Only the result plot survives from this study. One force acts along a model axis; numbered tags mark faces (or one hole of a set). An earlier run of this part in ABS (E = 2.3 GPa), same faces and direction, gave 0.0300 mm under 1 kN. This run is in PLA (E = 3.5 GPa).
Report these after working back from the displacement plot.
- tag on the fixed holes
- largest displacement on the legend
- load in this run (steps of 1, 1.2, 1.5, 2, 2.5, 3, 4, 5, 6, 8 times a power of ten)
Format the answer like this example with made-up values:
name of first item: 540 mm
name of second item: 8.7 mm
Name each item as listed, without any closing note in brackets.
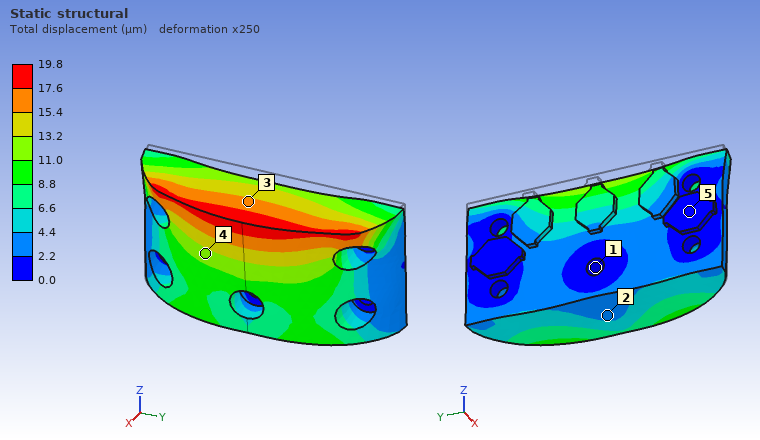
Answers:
tag on the fixed holes: 1
largest displacement on the legend: 19.8 µm
load in this run: 1 kN
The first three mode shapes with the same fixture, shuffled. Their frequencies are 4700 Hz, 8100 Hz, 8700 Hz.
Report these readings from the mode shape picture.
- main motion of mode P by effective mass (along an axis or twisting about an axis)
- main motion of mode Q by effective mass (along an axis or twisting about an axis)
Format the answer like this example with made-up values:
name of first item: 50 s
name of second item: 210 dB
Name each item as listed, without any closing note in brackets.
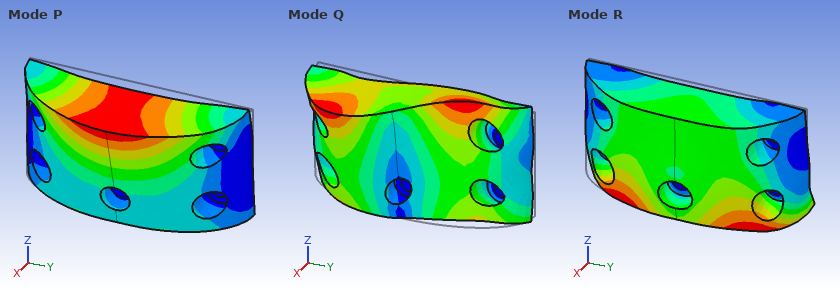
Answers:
main motion of mode P by effective mass: along X
main motion of mode Q by effective mass: along Y
